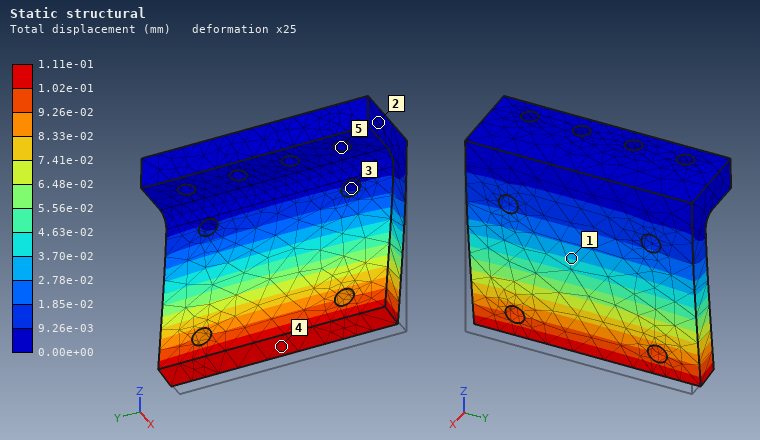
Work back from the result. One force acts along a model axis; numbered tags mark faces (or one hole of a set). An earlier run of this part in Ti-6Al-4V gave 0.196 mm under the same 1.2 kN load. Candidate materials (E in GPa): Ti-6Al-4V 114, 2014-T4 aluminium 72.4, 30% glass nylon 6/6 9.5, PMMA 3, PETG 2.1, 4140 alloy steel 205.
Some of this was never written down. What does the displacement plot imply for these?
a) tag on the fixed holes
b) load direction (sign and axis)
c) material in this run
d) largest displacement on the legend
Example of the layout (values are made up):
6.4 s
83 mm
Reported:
5
-X
4140 alloy steel
1.11e-01 mm
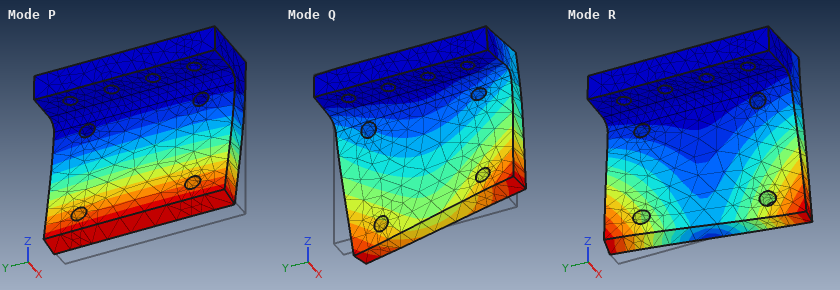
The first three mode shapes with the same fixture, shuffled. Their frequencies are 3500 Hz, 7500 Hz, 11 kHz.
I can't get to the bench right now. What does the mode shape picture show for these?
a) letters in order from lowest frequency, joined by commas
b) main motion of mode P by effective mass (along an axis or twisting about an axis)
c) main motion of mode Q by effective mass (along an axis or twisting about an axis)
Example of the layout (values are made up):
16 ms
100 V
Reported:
P, R, Q
along X
along Y
